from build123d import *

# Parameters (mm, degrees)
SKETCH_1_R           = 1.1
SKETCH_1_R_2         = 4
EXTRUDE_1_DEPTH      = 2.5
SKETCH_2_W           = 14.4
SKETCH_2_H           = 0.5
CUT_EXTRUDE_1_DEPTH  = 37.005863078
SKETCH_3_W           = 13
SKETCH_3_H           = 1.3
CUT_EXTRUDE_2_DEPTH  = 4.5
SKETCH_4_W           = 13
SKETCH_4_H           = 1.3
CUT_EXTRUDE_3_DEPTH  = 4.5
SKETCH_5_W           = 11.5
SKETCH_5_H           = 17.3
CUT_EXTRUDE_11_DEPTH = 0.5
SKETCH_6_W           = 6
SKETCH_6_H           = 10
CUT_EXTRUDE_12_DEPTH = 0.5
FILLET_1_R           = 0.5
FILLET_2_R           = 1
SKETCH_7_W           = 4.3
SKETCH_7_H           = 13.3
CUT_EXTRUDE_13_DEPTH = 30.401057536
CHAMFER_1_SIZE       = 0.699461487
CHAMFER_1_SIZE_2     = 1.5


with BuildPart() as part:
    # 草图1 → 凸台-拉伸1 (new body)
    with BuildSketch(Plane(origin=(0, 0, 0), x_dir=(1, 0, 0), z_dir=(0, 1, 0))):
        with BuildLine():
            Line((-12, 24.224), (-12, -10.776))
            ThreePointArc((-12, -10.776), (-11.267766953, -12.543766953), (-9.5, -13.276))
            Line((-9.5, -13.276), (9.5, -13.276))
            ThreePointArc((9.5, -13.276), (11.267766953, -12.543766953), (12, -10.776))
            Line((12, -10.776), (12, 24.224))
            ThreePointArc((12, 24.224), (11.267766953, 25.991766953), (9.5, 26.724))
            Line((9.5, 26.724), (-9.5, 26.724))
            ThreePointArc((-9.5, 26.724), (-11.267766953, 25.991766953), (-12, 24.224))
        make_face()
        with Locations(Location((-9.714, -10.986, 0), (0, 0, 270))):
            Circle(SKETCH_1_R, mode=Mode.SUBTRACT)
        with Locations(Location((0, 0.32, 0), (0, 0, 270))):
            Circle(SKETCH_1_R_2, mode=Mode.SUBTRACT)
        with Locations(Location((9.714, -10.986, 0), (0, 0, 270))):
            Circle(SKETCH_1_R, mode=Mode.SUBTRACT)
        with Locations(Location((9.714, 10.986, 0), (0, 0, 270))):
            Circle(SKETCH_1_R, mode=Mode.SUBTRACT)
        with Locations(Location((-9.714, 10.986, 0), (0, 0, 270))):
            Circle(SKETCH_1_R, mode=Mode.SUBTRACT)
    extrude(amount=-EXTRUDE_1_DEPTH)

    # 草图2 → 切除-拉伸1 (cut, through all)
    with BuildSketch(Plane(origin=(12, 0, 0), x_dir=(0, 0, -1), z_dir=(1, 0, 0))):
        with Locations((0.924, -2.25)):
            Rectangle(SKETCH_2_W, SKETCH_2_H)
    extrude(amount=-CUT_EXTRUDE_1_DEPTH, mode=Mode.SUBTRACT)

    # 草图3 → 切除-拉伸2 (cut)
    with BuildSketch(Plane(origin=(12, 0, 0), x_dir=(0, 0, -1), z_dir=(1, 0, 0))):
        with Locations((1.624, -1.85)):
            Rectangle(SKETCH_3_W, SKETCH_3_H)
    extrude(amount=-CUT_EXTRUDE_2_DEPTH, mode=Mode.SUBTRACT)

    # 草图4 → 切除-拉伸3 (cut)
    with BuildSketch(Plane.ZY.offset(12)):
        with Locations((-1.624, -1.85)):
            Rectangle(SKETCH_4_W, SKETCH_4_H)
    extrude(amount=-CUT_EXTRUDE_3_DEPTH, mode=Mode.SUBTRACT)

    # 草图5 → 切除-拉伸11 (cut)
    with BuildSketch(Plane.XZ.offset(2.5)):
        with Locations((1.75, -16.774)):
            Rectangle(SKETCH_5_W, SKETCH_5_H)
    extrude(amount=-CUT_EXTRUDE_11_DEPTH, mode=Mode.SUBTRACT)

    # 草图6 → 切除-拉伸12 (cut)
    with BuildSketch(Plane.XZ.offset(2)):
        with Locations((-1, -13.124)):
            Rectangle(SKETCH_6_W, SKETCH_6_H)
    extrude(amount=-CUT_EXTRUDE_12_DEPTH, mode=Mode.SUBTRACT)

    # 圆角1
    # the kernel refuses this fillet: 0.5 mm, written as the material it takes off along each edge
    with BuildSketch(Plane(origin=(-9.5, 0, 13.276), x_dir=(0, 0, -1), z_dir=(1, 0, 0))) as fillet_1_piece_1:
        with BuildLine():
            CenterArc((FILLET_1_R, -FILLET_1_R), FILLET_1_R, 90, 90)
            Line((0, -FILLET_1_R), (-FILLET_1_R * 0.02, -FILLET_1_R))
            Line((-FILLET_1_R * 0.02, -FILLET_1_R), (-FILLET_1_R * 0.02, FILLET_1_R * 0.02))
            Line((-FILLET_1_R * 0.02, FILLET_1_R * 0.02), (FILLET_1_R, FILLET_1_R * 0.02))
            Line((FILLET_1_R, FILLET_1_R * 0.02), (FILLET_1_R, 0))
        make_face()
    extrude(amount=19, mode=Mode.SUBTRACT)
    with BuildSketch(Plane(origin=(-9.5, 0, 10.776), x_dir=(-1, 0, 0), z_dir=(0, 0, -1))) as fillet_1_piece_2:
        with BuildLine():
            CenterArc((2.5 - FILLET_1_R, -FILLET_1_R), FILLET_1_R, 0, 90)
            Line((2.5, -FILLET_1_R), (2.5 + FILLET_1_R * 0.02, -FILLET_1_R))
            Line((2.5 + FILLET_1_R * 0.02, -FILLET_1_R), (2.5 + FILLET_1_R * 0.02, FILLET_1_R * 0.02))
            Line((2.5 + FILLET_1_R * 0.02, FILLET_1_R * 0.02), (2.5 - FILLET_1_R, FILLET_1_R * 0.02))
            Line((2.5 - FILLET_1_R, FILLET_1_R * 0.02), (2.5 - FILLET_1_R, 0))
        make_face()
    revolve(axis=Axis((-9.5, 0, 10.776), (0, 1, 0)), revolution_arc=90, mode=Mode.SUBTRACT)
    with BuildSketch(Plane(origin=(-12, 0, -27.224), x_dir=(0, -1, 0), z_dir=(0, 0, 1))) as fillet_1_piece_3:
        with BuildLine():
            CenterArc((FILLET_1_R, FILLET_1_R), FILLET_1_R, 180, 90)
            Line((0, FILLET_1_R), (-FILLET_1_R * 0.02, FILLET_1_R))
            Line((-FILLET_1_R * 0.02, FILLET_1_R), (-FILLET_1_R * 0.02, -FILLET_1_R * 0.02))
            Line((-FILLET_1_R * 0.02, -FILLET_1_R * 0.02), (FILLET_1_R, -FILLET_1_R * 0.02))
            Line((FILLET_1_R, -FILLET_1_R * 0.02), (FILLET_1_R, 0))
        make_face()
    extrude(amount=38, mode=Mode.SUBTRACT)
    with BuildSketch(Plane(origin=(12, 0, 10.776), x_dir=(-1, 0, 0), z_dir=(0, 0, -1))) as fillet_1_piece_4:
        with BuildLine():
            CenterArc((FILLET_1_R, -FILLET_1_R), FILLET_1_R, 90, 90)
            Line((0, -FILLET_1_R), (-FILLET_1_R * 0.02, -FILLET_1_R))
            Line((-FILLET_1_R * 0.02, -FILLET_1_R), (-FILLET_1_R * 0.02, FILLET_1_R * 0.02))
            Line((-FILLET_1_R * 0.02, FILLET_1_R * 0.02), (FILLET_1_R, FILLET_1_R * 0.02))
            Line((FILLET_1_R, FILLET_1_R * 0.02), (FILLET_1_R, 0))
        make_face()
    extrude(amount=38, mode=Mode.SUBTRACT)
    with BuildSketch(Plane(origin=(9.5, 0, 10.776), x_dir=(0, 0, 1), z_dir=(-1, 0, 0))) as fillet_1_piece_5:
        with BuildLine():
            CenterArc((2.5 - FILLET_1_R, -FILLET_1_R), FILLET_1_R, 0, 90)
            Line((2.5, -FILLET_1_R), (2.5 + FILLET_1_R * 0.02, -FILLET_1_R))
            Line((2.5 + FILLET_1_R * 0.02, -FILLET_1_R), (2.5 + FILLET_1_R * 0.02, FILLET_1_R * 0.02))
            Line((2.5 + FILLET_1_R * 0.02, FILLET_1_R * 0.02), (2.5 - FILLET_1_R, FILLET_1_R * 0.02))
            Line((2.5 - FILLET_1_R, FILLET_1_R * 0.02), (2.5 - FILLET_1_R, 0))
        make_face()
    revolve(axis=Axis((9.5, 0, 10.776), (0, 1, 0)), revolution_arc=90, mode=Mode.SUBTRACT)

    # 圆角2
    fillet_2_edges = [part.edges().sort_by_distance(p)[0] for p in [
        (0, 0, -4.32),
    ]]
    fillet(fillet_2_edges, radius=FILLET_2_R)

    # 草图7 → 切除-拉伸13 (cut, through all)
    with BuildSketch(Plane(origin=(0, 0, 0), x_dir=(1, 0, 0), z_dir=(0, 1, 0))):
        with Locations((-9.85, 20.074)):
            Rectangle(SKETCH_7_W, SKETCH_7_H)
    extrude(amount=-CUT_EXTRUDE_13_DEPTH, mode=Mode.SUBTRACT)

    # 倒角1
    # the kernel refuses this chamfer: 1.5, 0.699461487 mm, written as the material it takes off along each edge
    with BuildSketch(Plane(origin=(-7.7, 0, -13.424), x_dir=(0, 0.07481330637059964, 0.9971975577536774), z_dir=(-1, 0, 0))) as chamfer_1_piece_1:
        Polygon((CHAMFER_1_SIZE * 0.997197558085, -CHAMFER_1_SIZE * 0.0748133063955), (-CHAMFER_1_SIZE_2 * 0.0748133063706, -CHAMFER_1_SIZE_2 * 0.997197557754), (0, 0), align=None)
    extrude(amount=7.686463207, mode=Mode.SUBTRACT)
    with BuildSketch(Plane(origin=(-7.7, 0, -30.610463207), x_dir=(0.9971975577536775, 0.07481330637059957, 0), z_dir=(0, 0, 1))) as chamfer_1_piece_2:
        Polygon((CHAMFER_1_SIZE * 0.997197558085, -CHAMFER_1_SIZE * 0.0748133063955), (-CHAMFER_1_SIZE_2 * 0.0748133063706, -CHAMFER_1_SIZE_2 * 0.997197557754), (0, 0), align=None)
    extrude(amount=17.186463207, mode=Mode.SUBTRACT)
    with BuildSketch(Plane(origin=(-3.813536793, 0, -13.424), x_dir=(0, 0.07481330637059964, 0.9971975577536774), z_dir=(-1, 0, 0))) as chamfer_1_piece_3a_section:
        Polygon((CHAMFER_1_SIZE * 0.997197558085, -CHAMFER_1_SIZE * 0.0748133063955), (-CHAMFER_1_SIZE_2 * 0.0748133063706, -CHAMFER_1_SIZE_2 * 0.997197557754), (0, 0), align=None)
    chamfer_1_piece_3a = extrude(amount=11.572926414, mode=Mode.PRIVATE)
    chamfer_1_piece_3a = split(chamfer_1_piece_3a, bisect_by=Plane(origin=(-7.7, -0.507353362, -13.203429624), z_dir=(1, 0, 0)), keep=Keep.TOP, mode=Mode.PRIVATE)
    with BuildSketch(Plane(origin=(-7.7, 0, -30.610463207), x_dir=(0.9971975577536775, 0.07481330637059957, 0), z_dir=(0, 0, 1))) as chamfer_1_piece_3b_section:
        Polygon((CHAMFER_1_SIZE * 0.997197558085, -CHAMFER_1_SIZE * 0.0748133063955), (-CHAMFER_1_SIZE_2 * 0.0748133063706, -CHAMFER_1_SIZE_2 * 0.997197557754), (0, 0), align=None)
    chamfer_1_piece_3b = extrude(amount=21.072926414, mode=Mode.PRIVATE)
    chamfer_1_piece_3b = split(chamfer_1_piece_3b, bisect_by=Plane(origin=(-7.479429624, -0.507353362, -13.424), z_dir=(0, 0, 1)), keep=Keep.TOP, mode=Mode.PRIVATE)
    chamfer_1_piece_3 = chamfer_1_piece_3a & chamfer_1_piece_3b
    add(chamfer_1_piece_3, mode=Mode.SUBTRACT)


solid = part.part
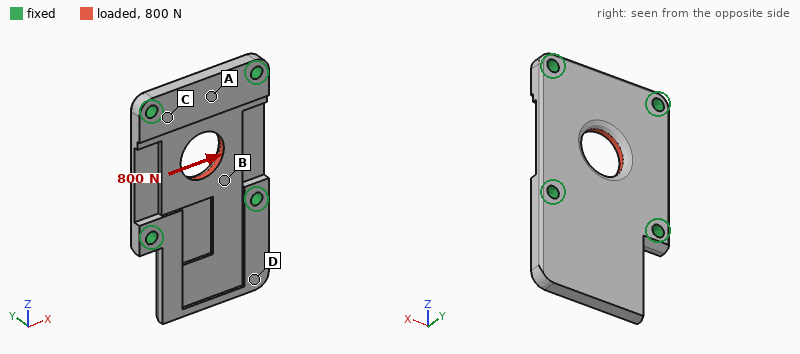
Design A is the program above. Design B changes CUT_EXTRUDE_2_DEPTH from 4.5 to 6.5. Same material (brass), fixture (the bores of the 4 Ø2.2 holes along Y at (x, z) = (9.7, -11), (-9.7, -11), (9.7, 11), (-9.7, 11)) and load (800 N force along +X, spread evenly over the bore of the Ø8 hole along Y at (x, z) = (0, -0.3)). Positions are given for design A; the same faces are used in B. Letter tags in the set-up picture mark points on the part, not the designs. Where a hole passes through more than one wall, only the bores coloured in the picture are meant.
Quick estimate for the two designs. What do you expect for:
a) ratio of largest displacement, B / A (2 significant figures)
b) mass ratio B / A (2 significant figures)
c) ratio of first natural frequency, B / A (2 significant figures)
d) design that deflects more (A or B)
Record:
1.3
0.99
1.00
B
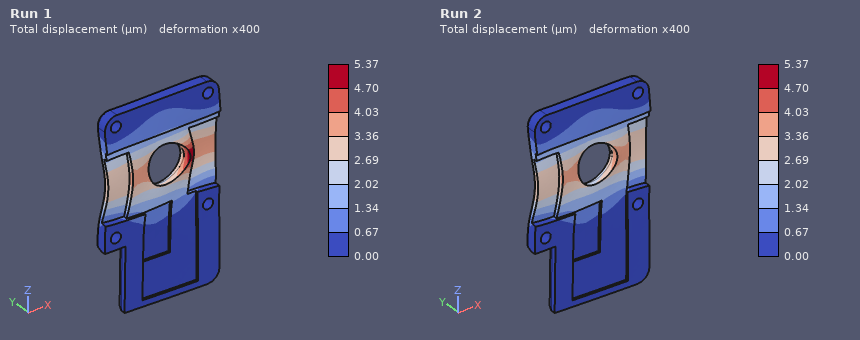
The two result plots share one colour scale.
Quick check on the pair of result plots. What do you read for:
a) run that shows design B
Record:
Run 1
